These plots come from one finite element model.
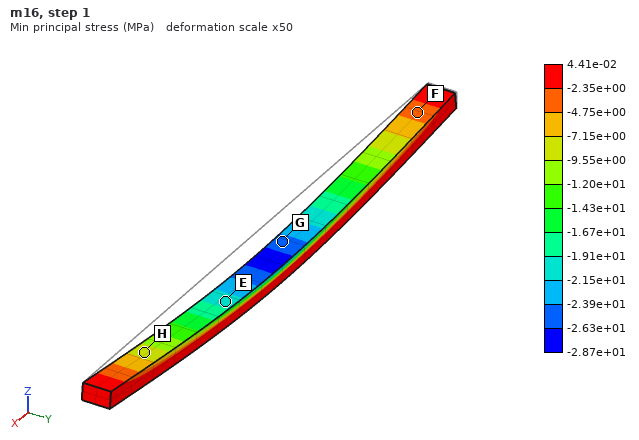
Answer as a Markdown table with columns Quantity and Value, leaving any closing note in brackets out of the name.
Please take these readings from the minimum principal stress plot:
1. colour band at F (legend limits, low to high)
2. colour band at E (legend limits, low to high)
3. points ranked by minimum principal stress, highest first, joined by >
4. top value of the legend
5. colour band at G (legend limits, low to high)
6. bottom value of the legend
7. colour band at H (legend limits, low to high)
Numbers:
| Quantity | Value |
|---|---|
| colour band at F | -4.75e+00 to -2.35e+00 MPa |
| colour band at E | -2.15e+01 to -1.91e+01 MPa |
| points ranked by minimum principal stress, highest first, joined by > | F > H > E > G |
| top value of the legend | 4.41e-02 MPa |
| colour band at G | -2.63e+01 to -2.39e+01 MPa |
| bottom value of the legend | -2.87e+01 MPa |
| colour band at H | -9.55e+00 to -7.15e+00 MPa |
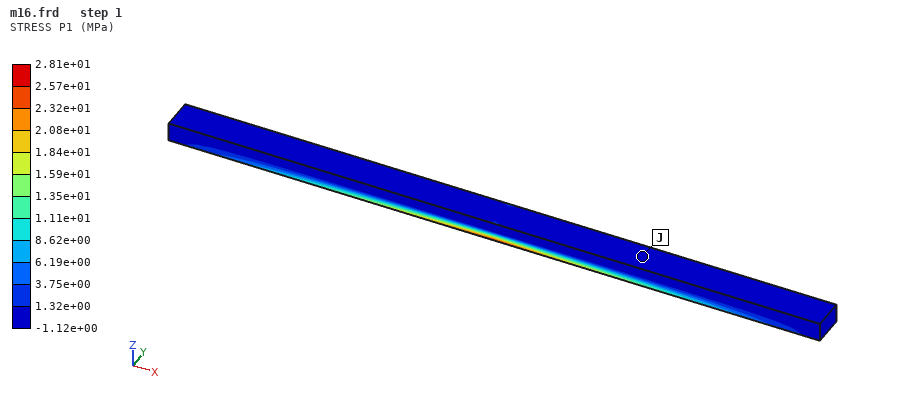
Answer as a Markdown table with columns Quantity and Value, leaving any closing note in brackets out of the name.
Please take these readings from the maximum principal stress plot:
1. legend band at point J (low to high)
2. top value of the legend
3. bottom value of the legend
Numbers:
| Quantity | Value |
|---|---|
| legend band at point J | -1.12e+00 to 1.32e+00 MPa |
| top value of the legend | 2.81e+01 MPa |
| bottom value of the legend | -1.12e+00 MPa |
